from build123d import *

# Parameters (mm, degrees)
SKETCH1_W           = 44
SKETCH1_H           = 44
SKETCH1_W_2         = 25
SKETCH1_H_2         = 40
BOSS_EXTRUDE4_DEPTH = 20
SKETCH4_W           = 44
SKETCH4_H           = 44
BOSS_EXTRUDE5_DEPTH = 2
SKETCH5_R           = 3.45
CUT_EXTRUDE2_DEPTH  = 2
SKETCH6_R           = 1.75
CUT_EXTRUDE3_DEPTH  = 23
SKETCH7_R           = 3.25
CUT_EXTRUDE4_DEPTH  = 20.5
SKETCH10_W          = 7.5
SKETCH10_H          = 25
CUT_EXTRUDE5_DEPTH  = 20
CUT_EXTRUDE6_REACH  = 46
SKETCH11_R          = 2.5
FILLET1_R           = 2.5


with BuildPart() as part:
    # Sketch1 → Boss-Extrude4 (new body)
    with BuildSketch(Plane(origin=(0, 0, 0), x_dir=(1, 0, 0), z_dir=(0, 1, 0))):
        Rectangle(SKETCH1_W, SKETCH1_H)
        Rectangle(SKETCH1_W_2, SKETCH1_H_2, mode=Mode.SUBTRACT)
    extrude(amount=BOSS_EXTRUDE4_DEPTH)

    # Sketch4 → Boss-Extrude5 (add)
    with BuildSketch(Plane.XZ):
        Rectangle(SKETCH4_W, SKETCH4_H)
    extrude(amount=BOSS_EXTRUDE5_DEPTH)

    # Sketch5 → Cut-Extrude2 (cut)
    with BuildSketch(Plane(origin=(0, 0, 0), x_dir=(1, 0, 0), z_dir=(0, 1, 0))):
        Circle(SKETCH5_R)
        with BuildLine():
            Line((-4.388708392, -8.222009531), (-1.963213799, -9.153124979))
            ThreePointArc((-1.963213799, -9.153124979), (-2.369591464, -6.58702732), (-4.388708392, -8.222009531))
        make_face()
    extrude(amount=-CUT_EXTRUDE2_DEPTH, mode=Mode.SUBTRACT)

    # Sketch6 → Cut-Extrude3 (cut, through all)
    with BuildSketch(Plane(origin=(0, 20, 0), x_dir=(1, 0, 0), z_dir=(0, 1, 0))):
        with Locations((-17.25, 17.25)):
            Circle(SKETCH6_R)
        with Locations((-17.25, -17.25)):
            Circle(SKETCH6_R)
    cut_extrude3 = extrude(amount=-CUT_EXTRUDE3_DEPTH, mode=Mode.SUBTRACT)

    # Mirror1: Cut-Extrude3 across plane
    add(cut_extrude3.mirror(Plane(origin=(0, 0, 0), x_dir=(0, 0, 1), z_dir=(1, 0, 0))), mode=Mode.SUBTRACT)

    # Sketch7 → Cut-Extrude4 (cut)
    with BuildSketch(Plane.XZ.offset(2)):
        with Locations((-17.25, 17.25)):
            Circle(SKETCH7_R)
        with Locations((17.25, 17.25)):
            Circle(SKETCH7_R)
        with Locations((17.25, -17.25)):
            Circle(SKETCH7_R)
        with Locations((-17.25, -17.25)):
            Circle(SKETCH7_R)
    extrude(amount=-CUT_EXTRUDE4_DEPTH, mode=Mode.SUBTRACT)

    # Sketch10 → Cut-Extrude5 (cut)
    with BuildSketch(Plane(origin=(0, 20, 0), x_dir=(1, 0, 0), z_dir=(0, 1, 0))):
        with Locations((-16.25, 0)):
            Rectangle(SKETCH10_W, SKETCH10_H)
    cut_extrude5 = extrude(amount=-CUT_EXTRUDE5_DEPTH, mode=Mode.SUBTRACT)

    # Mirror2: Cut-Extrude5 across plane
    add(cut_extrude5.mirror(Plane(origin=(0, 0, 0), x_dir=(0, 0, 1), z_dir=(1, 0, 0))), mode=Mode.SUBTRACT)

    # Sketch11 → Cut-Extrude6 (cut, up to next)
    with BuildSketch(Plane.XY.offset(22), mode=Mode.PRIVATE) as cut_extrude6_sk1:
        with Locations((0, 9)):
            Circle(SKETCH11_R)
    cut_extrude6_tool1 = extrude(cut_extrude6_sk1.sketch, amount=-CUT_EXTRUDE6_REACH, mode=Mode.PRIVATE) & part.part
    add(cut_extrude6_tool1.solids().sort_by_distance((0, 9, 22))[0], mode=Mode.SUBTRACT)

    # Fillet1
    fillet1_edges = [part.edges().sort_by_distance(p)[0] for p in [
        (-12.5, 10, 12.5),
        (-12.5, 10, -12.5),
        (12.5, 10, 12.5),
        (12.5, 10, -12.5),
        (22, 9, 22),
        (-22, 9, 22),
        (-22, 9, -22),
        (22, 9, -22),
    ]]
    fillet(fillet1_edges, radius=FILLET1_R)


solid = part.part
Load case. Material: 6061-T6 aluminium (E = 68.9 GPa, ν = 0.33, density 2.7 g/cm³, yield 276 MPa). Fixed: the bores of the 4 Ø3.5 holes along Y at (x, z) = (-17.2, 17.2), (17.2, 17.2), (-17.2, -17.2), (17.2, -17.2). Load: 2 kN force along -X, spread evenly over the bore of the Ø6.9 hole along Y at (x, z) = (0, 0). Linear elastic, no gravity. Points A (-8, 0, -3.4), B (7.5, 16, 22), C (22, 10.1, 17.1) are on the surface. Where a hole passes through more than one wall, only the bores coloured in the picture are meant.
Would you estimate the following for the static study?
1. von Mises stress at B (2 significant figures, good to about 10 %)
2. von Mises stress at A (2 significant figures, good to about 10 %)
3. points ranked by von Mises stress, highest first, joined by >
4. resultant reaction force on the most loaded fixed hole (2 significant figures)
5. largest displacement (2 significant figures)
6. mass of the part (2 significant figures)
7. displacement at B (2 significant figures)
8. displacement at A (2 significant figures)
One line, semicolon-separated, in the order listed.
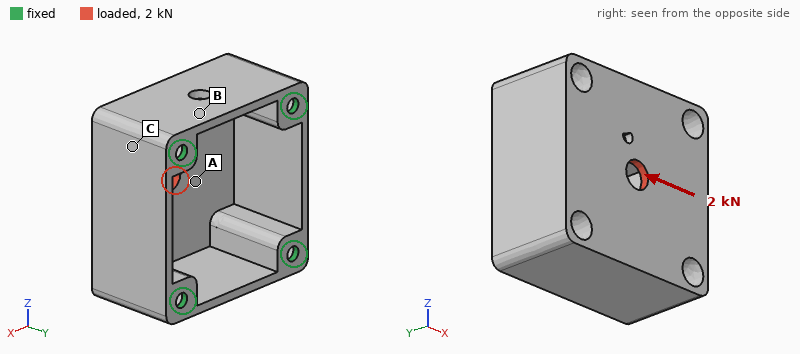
18 MPa; 35 MPa; A > B > C; 770 N; 36 µm; 32 g; 8.9 µm; 33 µm
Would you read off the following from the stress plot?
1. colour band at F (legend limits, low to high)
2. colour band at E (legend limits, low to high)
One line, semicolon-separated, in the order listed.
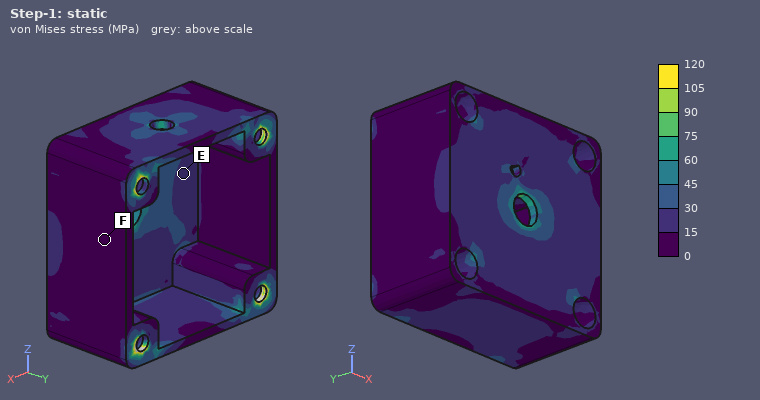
0 to 15 MPa; 15 to 30 MPa
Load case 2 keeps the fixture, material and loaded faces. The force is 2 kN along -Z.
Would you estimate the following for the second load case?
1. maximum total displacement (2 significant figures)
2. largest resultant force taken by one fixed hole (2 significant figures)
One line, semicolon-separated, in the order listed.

36 µm; 750 N
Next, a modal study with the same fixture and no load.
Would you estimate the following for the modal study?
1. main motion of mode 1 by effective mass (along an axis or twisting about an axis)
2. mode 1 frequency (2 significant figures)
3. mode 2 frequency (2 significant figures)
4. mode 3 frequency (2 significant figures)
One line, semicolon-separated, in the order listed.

along Y; 9300 Hz; 10 kHz; 10 kHz
